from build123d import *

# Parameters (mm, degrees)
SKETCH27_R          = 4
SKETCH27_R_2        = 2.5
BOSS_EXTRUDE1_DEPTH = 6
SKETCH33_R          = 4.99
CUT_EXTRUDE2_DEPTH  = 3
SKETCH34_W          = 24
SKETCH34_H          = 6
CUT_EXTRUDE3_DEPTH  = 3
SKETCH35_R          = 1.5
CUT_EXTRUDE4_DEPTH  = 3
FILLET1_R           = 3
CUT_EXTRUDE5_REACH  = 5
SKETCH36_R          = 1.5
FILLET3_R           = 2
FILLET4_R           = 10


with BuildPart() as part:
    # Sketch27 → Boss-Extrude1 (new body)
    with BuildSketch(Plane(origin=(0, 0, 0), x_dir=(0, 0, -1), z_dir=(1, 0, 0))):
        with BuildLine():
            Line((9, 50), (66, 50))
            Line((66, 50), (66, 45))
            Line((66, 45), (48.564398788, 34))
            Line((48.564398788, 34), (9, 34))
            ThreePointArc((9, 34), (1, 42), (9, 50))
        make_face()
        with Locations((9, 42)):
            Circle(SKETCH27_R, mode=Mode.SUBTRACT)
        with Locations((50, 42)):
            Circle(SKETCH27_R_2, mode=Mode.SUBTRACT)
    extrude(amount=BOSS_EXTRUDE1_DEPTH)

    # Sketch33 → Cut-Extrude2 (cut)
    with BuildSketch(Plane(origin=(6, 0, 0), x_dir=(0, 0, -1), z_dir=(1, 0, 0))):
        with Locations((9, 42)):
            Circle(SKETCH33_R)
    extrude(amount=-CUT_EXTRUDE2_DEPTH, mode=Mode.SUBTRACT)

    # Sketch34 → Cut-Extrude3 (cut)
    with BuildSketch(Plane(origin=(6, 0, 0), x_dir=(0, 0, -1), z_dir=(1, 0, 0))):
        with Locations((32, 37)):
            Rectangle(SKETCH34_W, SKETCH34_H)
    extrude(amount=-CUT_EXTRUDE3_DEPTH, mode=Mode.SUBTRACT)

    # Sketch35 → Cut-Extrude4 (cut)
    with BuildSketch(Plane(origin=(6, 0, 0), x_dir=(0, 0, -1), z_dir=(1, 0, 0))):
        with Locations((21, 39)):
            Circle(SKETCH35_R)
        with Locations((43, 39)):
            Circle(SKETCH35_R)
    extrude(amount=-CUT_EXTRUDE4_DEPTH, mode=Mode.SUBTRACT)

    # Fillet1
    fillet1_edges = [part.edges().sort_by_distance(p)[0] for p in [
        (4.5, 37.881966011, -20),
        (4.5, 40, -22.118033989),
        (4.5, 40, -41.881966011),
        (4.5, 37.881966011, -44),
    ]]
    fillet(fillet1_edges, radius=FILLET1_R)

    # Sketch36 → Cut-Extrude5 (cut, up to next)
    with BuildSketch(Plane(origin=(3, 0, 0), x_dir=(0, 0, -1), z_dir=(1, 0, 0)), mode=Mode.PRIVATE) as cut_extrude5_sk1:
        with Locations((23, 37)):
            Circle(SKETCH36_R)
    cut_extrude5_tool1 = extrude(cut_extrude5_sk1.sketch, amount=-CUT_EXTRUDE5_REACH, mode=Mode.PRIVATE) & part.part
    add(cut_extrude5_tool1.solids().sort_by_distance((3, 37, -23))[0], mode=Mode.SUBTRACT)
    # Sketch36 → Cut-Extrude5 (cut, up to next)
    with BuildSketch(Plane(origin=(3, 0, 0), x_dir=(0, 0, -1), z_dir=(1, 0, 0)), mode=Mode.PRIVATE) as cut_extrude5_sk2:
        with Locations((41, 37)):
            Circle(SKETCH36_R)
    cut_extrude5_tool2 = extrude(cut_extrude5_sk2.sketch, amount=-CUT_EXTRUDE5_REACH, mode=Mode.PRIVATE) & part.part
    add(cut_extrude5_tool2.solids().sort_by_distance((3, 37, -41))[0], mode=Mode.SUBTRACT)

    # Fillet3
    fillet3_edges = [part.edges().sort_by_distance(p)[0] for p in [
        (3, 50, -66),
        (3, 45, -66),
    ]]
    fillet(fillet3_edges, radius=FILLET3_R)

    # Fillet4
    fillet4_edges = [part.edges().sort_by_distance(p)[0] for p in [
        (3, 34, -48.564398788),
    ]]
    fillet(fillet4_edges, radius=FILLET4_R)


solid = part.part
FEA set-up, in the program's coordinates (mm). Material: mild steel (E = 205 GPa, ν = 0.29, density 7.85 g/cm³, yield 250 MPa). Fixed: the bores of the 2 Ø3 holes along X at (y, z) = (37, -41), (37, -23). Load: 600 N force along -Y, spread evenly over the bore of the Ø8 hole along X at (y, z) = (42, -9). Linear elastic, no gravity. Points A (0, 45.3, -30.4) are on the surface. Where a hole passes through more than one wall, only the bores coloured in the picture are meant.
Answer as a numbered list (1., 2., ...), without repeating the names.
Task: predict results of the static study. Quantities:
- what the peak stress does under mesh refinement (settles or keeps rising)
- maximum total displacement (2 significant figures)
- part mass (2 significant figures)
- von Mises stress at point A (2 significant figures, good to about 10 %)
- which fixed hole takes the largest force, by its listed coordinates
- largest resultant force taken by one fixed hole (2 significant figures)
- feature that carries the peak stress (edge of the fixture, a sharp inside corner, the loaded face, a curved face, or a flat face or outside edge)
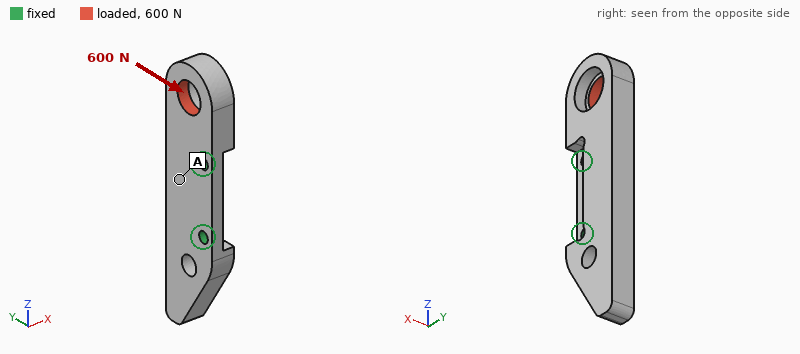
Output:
1. keeps rising
2. 14 µm
3. 35 g
4. 19 MPa
5. (37, -23)
6. 1.0 kN
7. edge of the fixture
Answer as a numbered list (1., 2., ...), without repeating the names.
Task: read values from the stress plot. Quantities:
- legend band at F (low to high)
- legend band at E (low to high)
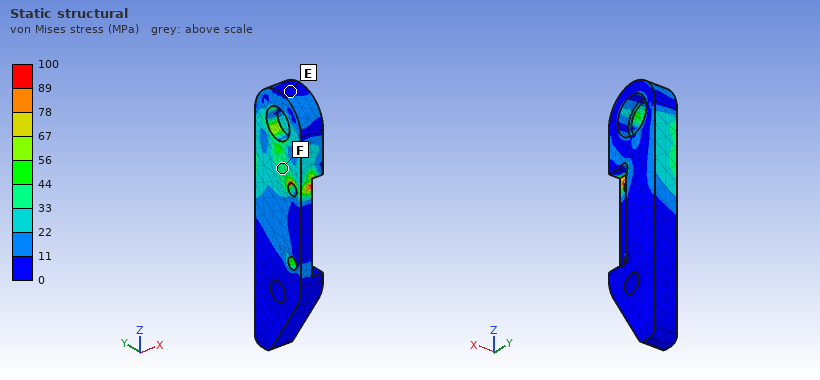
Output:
1. 33 to 44 MPa
2. 0 to 11 MPa
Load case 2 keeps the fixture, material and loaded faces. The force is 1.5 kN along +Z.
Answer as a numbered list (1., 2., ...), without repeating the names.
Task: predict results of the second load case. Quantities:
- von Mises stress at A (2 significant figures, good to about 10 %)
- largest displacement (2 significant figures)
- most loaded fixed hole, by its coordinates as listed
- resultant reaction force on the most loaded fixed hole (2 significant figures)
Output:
1. 21 MPa
2. 13 µm
3. (37, -23)
4. 1.2 kN
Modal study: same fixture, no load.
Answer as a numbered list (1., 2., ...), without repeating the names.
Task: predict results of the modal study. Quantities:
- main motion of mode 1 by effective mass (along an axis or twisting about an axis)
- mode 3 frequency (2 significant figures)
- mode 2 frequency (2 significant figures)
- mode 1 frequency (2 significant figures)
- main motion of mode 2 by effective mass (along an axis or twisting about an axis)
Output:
1. along X
2. 10 kHz
3. 7100 Hz
4. 5600 Hz
5. along X
